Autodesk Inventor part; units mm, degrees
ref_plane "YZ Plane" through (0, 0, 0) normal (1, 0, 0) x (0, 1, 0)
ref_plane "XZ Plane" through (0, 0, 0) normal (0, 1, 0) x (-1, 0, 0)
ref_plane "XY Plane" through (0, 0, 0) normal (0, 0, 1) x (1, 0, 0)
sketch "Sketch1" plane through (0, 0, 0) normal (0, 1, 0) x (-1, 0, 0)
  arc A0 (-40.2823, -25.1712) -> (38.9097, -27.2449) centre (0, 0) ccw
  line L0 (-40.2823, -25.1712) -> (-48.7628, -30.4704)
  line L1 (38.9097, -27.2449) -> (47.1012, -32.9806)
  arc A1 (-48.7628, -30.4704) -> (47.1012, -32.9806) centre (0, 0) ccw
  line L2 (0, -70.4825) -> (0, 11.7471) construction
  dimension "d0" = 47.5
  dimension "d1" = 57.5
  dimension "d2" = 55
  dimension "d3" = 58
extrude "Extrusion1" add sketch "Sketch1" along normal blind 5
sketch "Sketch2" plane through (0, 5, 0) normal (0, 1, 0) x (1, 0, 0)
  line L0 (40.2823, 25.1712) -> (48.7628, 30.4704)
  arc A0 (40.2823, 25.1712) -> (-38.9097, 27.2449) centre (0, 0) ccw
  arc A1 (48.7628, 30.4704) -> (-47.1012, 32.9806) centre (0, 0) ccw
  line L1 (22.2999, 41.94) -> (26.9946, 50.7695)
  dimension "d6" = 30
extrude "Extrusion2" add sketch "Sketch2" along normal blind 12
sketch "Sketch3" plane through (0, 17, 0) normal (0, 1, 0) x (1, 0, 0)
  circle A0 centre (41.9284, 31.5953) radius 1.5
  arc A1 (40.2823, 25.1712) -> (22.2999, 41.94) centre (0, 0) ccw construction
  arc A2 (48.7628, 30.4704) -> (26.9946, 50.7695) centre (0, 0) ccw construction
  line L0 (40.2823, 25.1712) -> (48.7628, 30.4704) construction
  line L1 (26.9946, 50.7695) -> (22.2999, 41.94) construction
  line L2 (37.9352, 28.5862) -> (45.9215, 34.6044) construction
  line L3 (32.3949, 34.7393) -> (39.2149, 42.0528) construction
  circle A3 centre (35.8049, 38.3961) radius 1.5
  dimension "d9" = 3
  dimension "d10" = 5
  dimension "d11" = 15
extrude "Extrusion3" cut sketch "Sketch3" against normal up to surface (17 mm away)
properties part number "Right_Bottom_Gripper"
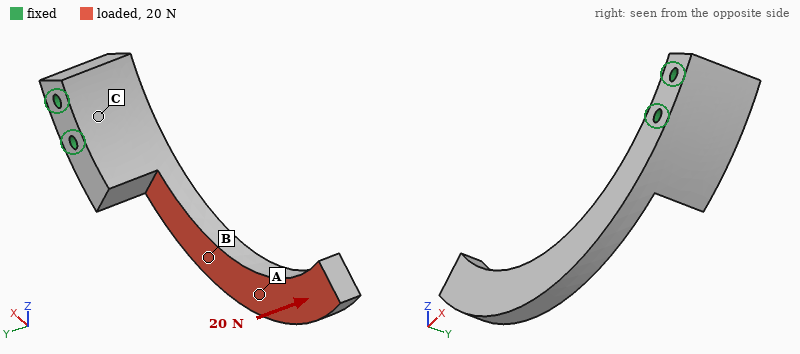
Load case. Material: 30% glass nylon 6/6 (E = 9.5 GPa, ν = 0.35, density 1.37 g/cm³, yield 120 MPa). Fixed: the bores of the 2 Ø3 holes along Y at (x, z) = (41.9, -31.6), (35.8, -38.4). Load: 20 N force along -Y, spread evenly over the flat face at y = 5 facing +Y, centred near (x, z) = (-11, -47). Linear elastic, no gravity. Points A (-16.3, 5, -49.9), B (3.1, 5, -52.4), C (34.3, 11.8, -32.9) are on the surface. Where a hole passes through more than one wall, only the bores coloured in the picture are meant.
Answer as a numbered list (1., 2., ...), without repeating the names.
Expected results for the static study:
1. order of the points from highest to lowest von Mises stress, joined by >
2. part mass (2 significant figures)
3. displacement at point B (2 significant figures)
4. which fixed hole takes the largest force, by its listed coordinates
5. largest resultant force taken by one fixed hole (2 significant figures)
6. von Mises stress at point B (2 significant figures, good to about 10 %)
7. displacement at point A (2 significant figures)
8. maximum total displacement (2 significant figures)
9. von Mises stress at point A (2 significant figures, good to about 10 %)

1. B > A > C
2. 11 g
3. 0.20 mm
4. (35.8, -38.4)
5. 25 N
6. 8.5 MPa
7. 0.53 mm
8. 1.2 mm
9. 3.6 MPa
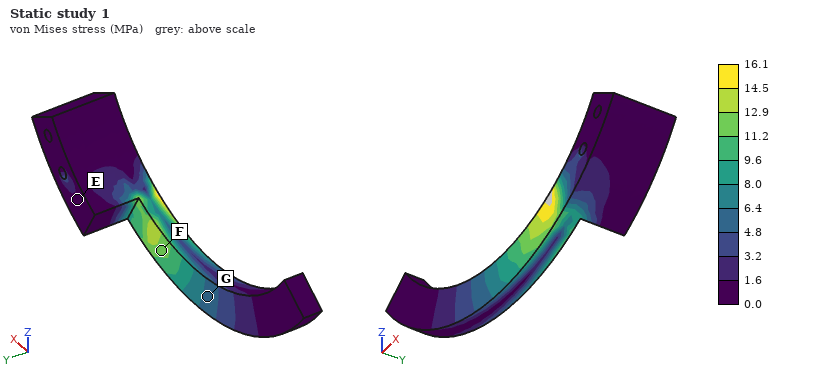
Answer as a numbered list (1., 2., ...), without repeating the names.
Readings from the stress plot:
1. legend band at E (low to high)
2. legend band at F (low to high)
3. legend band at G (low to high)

1. 0.0 to 1.6 MPa
2. 11.2 to 12.9 MPa
3. 4.8 to 6.4 MPa
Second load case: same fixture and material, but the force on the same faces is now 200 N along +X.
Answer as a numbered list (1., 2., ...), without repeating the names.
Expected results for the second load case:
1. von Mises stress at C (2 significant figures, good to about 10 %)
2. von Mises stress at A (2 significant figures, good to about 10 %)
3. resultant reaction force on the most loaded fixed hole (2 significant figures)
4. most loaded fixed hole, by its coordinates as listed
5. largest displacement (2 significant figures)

1. 2.3 MPa
2. 7.1 MPa
3. 270 N
4. (35.8, -38.4)
5. 1.0 mm
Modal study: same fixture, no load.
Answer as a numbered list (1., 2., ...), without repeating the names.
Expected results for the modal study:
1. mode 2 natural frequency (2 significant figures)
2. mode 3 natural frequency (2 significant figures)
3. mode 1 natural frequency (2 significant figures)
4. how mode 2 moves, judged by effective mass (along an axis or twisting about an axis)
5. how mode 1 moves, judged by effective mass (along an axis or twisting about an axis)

1. 620 Hz
2. 1700 Hz
3. 360 Hz
4. along Z
5. along Y
